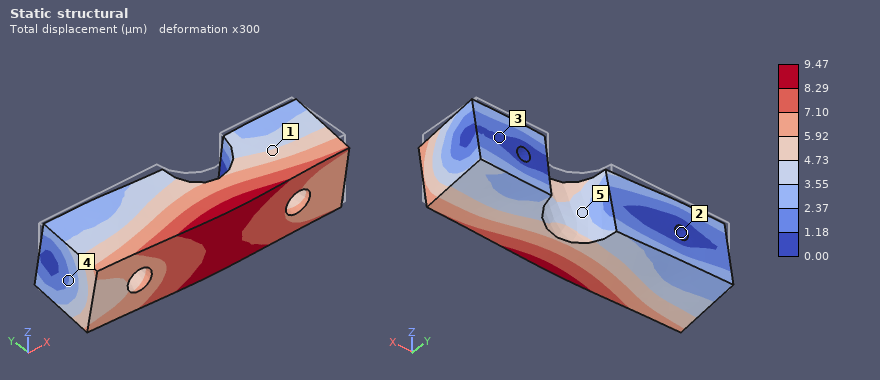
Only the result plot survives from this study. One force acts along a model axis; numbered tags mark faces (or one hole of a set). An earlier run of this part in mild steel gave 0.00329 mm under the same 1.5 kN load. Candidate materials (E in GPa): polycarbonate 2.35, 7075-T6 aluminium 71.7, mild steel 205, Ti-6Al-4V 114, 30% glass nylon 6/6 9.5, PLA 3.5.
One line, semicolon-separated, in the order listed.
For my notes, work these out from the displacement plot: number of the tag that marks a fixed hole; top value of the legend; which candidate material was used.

2; 9.47 µm; 7075-T6 aluminium
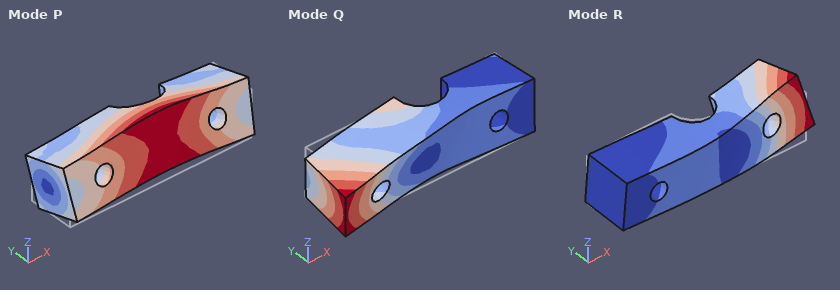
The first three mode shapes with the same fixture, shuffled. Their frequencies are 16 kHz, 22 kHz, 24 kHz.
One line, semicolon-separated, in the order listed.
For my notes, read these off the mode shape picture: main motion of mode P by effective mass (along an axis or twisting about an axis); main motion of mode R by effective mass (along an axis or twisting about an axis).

along Z; twisting about Y
